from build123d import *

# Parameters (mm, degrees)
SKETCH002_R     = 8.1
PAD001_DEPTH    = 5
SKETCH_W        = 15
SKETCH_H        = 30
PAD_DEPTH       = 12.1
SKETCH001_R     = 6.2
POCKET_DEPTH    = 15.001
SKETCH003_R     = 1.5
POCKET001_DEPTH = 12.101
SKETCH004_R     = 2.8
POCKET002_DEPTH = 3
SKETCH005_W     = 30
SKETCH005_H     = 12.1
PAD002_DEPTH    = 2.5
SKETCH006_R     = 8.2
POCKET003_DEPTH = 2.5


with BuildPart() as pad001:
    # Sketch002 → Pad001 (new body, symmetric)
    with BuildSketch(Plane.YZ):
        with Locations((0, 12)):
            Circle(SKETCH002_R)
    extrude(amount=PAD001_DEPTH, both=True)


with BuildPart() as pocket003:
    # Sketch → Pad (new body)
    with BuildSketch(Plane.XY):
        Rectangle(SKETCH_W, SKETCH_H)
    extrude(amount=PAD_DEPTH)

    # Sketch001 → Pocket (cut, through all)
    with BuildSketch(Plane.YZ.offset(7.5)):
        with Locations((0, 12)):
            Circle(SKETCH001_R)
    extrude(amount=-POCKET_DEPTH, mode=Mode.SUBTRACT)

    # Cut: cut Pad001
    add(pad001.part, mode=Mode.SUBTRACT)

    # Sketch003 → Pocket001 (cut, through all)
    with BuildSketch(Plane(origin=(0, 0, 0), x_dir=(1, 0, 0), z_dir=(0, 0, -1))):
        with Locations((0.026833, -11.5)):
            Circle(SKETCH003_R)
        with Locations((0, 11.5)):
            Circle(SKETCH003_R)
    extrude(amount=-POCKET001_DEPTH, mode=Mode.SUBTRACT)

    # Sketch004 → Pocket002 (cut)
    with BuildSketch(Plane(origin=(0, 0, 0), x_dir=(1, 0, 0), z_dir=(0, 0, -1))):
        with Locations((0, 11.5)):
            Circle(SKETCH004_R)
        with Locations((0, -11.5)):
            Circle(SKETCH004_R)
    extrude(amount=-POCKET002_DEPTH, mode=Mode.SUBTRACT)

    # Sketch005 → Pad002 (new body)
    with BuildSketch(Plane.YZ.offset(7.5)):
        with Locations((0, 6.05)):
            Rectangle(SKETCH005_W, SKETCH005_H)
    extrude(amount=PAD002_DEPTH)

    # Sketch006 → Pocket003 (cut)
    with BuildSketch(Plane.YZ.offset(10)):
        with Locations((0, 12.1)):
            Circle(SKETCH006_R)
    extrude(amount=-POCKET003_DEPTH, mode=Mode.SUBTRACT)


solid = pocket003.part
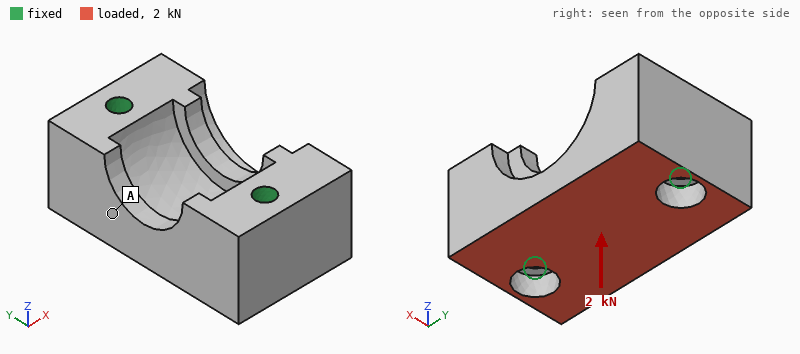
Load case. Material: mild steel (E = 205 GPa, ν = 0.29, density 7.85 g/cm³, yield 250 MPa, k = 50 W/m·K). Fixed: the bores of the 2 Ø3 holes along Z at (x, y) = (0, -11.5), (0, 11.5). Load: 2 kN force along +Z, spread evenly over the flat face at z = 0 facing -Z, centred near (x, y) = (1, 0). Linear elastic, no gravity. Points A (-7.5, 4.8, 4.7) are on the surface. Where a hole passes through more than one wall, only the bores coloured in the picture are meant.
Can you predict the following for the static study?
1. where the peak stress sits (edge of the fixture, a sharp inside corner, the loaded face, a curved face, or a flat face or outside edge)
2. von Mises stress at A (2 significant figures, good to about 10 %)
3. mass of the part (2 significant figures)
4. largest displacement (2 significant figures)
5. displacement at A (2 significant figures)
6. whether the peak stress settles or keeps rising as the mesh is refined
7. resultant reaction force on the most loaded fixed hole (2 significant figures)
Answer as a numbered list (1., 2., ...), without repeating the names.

1. edge of the fixture
2. 5.9 MPa
3. 35 g
4. 2.0 µm
5. 0.72 µm
6. keeps rising
7. 1.1 kN
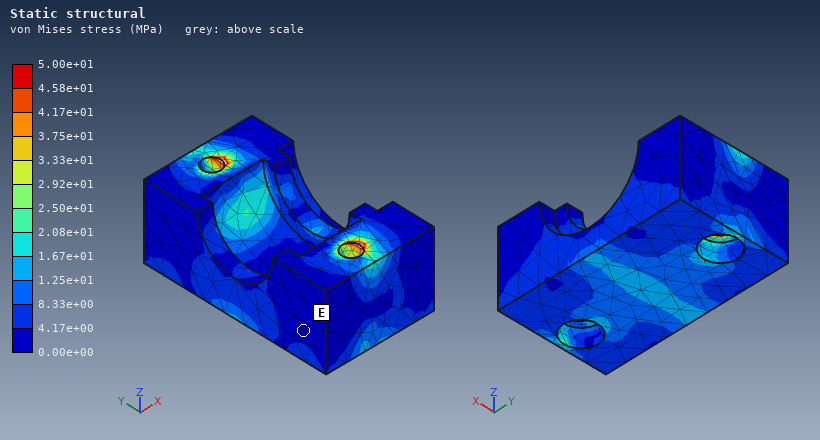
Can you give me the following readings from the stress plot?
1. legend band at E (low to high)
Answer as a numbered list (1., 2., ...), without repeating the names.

1. 0.00e+00 to 4.17e+00 MPa
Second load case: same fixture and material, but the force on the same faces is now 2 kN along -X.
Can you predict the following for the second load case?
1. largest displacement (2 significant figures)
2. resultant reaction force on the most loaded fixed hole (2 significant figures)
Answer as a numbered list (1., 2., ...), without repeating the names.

1. 4.0 µm
2. 1.0 kN
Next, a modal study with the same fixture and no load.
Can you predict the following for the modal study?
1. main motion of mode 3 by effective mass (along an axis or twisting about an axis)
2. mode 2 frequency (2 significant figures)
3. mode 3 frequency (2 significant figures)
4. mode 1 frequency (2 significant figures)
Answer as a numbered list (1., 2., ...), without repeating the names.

1. along Z
2. 44 kHz
3. 47 kHz
4. 33 kHz
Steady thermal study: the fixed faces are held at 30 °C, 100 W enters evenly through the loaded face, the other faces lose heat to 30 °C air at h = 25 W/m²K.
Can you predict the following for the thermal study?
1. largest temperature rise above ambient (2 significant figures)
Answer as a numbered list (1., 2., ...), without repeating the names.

1. 75 K
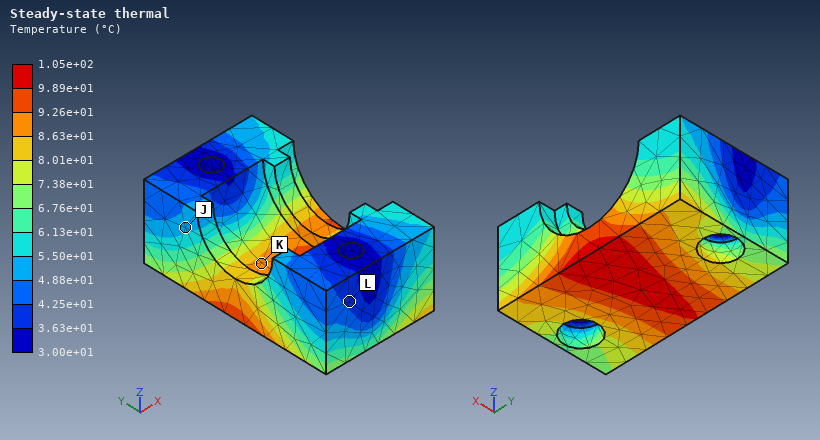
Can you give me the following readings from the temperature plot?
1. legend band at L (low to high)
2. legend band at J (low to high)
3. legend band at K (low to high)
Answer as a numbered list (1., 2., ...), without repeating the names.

1. 3.63e+01 to 4.25e+01 °C
2. 4.88e+01 to 5.50e+01 °C
3. 8.63e+01 to 9.26e+01 °C
